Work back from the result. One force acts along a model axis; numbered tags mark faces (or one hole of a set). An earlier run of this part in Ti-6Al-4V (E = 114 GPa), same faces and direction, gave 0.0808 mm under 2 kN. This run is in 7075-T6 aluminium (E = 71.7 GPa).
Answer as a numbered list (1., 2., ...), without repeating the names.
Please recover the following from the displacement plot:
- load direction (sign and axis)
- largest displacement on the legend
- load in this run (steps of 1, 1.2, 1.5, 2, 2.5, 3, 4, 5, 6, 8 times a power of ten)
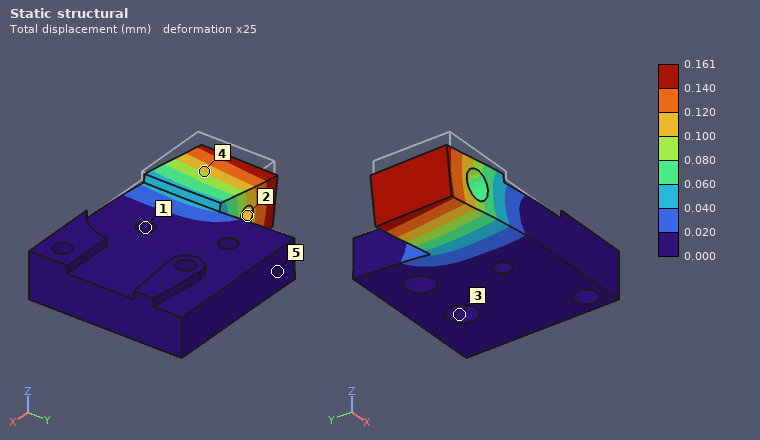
1. -Z
2. 0.161 mm
3. 2.5 kN
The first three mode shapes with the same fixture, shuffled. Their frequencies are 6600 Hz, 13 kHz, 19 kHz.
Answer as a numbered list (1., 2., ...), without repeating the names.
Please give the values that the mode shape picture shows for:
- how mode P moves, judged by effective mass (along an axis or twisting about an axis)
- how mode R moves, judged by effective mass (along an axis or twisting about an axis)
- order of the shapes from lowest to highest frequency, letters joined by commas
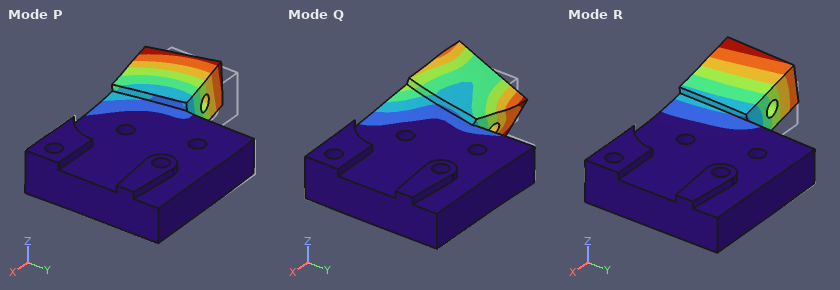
1. along Y
2. along Z
3. R, P, Q
